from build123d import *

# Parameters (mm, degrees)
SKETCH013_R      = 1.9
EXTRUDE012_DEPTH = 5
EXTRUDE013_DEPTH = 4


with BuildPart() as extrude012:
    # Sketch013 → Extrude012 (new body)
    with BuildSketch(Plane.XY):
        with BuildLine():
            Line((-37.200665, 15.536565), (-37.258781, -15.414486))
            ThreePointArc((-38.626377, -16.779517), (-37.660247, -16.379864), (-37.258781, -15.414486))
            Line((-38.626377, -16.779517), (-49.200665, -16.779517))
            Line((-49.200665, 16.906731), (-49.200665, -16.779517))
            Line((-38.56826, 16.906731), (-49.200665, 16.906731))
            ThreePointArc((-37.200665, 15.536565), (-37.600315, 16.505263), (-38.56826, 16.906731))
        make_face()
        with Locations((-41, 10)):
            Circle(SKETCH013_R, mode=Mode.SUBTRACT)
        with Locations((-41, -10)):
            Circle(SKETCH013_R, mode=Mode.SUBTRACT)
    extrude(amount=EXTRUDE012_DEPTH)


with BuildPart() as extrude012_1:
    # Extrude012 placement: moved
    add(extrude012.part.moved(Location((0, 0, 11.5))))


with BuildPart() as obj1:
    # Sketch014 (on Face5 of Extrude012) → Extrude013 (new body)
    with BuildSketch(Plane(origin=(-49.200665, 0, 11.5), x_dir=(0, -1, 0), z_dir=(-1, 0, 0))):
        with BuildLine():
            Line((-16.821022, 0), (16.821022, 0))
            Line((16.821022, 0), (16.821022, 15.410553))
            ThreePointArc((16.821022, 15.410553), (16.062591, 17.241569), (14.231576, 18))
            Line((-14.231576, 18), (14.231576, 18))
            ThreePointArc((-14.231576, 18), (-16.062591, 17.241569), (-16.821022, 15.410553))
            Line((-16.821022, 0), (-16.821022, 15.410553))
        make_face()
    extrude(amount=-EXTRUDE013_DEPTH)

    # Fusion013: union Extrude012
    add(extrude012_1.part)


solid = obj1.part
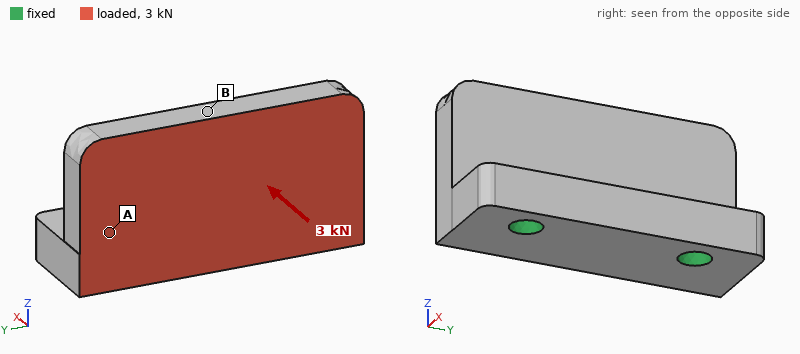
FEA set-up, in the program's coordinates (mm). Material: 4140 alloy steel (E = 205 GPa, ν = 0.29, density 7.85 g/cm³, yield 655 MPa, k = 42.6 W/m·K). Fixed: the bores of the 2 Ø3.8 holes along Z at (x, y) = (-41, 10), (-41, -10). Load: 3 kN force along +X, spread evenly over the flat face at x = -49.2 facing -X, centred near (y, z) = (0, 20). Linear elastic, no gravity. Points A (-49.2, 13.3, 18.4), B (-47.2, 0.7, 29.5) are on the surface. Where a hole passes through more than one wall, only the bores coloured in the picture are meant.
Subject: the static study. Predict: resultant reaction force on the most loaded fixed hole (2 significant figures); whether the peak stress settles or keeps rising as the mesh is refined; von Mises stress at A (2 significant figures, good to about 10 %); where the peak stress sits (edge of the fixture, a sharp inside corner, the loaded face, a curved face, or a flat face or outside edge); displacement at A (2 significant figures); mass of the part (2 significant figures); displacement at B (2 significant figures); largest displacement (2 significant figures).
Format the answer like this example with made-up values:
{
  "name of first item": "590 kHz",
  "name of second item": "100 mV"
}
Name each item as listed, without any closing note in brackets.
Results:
{
  "resultant reaction force on the most loaded fixed hole": "1.5 kN",
  "whether the peak stress settles or keeps rising as the mesh is refined": "keeps rising",
  "von Mises stress at A": "110 MPa",
  "where the peak stress sits": "edge of the fixture",
  "displacement at A": "15 µm",
  "mass of the part": "29 g",
  "displacement at B": "51 µm",
  "largest displacement": "52 µm"
}
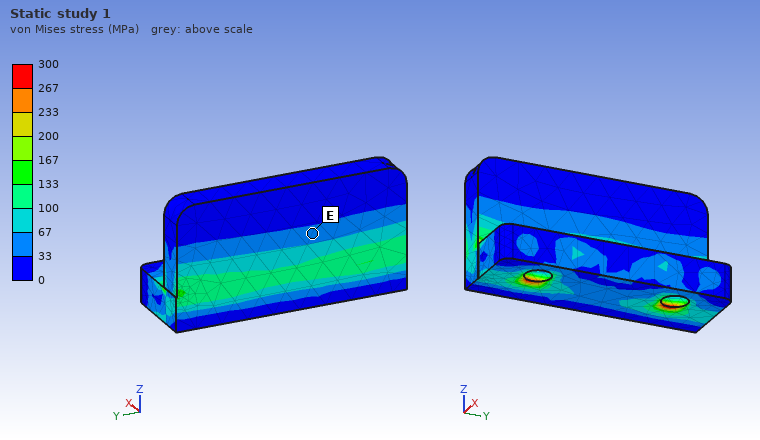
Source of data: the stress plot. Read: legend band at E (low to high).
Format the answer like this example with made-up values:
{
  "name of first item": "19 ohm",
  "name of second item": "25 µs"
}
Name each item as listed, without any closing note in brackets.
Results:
{
  "legend band at E": "33 to 67 MPa"
}
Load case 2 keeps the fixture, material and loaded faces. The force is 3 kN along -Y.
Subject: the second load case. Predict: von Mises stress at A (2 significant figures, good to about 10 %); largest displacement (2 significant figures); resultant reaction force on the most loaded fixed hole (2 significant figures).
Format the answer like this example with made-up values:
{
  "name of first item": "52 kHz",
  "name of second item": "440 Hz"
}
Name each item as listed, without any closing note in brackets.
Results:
{
  "von Mises stress at A": "22 MPa",
  "largest displacement": "8.3 µm",
  "resultant reaction force on the most loaded fixed hole": "2.0 kN"
}
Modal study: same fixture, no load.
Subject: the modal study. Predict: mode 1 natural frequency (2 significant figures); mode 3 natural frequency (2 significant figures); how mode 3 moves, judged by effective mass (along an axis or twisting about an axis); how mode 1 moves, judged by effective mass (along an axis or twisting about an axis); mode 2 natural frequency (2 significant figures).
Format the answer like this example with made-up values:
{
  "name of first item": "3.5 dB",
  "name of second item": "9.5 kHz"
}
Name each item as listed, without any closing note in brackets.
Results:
{
  "mode 1 natural frequency": "11 kHz",
  "mode 3 natural frequency": "26 kHz",
  "how mode 3 moves, judged by effective mass": "along Y",
  "how mode 1 moves, judged by effective mass": "along X",
  "mode 2 natural frequency": "17 kHz"
}
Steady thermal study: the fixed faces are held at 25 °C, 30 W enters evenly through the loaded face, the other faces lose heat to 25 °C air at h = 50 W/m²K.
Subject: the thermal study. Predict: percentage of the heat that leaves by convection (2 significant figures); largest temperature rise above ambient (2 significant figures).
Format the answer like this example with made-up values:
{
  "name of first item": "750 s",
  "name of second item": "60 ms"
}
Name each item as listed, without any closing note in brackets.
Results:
{
  "percentage of the heat that leaves by convection": "6.8 %",
  "largest temperature rise above ambient": "54 K"
}
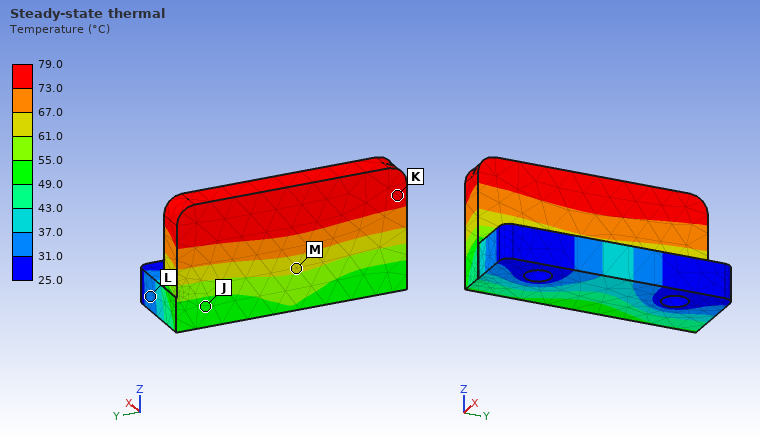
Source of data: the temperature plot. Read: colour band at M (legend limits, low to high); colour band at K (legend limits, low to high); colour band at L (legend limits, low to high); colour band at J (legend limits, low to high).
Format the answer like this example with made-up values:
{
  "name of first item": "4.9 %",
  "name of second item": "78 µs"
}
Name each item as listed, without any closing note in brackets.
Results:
{
  "colour band at M": "61.0 to 67.0 °C",
  "colour band at K": "73.0 to 79.0 °C",
  "colour band at L": "31.0 to 37.0 °C",
  "colour band at J": "49.0 to 55.0 °C"
}
